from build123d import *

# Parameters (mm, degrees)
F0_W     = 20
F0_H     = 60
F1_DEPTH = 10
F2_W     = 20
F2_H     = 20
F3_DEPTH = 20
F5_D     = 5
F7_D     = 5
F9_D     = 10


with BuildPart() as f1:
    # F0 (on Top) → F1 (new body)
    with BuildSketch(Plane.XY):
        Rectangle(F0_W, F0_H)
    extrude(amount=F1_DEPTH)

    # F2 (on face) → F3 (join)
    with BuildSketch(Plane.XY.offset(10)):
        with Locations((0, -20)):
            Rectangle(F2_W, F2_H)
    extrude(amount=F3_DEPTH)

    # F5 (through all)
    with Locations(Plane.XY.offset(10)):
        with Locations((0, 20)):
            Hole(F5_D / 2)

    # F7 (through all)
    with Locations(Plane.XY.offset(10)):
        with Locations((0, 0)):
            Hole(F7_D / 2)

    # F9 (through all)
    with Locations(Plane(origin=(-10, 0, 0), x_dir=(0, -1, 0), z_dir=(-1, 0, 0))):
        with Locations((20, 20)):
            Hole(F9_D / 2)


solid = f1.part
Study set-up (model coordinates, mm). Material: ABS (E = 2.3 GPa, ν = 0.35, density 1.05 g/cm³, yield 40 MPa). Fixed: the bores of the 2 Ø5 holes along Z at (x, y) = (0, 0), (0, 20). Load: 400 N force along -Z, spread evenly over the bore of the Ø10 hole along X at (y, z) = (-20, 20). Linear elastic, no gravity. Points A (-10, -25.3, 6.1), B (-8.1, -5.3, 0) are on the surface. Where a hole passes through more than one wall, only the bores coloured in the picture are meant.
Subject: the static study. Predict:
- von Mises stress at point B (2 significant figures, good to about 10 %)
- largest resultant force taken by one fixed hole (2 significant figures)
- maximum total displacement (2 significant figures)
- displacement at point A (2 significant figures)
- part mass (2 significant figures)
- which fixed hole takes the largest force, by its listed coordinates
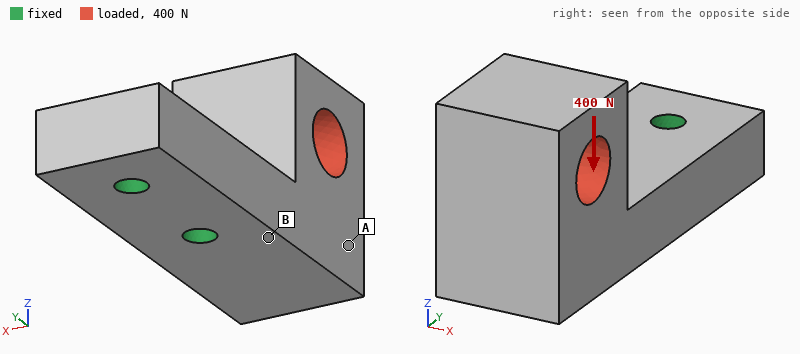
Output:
13 MPa
490 N
0.74 mm
0.43 mm
19 g
(0, 0)
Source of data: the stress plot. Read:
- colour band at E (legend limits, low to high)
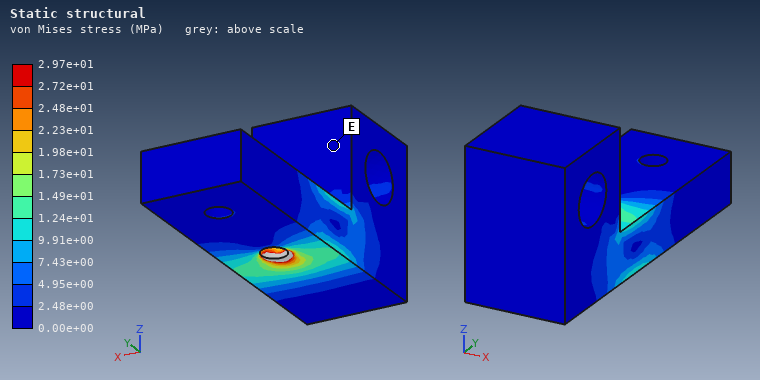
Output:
0.00e+00 to 2.48e+00 MPa
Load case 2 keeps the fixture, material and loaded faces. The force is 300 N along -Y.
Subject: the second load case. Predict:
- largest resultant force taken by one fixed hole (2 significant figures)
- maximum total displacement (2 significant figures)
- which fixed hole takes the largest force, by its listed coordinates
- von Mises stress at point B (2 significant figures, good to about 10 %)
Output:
270 N
0.63 mm
(0, 0)
9.9 MPa
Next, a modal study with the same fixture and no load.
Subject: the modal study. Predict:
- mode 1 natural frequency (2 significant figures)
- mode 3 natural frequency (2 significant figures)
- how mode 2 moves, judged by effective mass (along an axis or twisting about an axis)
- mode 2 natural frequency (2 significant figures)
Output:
1200 Hz
2900 Hz
along X
1600 Hz
